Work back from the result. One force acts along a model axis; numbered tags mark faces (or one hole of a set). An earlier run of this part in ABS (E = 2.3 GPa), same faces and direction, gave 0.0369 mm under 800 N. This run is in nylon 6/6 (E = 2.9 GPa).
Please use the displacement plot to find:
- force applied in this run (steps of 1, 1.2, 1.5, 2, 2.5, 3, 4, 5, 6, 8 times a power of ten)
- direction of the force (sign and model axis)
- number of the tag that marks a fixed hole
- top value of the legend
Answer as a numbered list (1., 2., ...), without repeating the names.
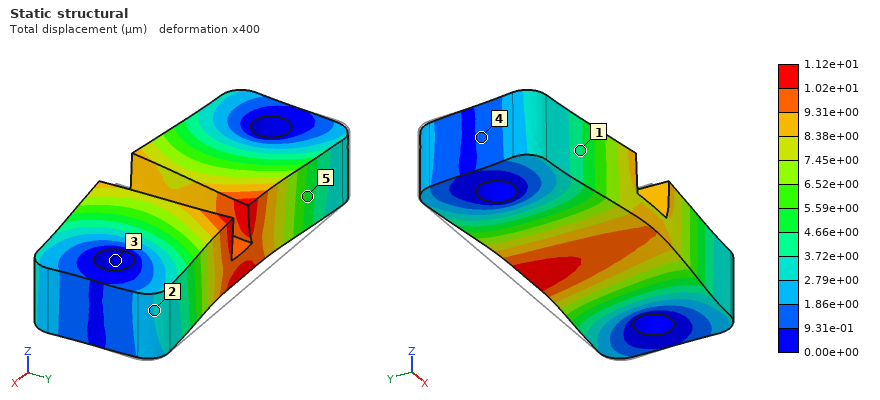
1. 300 N
2. -Y
3. 3
4. 1.12e+01 µm
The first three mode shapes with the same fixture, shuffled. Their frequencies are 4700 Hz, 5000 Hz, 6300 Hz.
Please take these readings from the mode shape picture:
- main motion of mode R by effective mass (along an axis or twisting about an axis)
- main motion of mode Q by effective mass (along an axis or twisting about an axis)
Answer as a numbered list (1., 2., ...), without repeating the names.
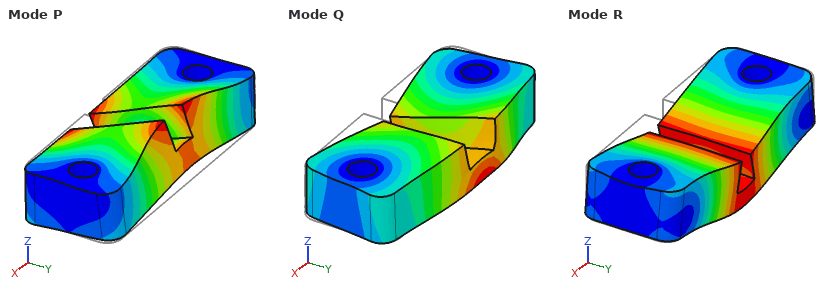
1. along Z
2. along Y
